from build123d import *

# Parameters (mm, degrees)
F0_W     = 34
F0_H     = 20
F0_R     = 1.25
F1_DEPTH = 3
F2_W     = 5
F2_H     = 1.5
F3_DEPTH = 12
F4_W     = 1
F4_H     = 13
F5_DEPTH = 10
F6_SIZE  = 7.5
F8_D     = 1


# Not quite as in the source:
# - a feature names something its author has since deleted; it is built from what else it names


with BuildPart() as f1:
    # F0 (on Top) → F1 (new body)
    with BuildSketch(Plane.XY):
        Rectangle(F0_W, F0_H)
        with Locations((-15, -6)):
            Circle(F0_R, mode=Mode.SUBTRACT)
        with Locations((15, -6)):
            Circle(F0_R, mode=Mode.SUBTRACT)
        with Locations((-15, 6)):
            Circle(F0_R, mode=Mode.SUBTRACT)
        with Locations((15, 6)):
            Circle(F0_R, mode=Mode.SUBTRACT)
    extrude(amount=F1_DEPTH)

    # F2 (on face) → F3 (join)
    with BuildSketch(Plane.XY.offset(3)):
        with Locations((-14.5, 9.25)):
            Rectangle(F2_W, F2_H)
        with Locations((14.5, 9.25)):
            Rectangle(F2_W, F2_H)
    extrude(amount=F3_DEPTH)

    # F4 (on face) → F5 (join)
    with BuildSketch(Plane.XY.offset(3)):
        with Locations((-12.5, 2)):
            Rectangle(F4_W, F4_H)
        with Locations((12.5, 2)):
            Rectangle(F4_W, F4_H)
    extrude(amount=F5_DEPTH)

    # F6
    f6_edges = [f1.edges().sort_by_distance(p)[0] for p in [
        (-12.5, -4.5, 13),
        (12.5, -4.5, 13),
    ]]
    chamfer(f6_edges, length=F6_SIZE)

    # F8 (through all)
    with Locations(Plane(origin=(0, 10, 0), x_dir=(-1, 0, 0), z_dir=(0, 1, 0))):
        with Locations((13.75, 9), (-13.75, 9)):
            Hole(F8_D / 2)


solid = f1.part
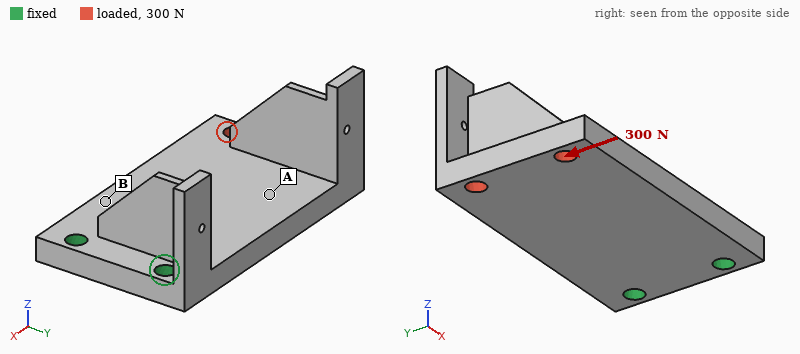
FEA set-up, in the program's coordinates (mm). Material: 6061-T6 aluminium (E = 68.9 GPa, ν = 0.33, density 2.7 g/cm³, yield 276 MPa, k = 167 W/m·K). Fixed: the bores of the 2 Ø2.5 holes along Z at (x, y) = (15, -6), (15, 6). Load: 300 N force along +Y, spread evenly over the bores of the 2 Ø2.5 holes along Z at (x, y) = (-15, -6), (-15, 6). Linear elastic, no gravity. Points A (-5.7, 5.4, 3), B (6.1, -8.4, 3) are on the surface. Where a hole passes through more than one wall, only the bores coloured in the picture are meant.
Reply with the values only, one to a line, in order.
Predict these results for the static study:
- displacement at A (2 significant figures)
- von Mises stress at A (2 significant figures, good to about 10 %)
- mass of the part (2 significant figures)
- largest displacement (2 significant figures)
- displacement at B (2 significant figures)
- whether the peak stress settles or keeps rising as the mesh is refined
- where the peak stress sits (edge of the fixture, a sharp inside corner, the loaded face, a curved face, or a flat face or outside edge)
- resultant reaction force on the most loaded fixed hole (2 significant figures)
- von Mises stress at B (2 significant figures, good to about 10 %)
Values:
18 µm
12 MPa
6.4 g
34 µm
7.6 µm
keeps rising
edge of the fixture
680 N
26 MPa
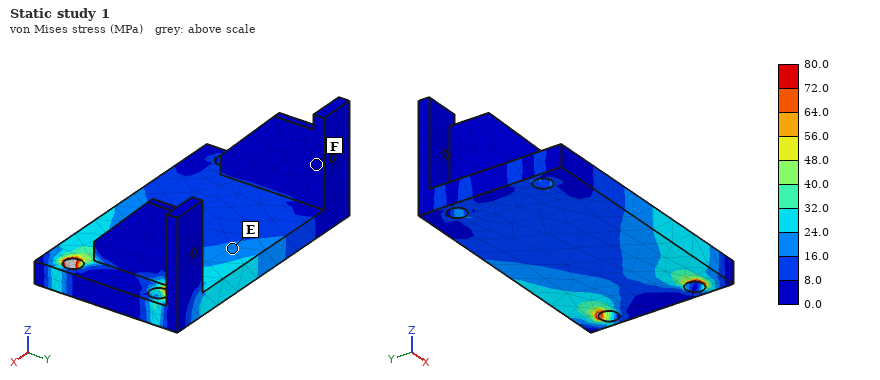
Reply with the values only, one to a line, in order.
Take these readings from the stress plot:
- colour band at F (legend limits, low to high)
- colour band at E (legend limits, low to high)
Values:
0.0 to 8.0 MPa
16.0 to 24.0 MPa
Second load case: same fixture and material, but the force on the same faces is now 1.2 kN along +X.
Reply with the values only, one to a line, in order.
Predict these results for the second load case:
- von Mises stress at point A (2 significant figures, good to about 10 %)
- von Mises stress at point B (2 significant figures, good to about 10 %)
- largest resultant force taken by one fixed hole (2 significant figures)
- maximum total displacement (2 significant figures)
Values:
20 MPa
20 MPa
610 N
13 µm
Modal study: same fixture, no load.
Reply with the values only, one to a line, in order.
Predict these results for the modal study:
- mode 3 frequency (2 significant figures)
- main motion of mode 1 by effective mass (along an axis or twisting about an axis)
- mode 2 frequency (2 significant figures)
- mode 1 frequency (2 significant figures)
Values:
9800 Hz
along Z
6300 Hz
2100 Hz
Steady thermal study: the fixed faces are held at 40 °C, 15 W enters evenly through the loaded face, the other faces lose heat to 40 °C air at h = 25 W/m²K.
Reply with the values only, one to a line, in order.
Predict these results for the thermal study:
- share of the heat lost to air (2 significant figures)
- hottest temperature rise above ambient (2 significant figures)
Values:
8.3 %
47 K
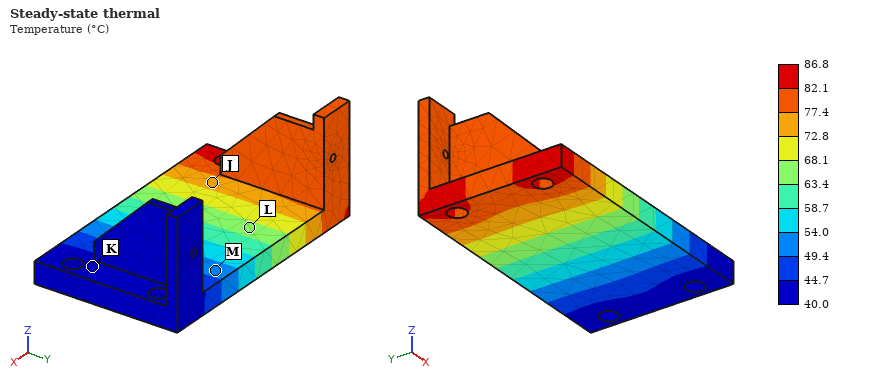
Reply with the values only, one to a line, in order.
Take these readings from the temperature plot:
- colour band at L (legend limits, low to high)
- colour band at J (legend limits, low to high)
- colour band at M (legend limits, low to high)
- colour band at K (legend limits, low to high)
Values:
63.4 to 68.1 °C
72.8 to 77.4 °C
49.4 to 54.0 °C
40.0 to 44.7 °C
